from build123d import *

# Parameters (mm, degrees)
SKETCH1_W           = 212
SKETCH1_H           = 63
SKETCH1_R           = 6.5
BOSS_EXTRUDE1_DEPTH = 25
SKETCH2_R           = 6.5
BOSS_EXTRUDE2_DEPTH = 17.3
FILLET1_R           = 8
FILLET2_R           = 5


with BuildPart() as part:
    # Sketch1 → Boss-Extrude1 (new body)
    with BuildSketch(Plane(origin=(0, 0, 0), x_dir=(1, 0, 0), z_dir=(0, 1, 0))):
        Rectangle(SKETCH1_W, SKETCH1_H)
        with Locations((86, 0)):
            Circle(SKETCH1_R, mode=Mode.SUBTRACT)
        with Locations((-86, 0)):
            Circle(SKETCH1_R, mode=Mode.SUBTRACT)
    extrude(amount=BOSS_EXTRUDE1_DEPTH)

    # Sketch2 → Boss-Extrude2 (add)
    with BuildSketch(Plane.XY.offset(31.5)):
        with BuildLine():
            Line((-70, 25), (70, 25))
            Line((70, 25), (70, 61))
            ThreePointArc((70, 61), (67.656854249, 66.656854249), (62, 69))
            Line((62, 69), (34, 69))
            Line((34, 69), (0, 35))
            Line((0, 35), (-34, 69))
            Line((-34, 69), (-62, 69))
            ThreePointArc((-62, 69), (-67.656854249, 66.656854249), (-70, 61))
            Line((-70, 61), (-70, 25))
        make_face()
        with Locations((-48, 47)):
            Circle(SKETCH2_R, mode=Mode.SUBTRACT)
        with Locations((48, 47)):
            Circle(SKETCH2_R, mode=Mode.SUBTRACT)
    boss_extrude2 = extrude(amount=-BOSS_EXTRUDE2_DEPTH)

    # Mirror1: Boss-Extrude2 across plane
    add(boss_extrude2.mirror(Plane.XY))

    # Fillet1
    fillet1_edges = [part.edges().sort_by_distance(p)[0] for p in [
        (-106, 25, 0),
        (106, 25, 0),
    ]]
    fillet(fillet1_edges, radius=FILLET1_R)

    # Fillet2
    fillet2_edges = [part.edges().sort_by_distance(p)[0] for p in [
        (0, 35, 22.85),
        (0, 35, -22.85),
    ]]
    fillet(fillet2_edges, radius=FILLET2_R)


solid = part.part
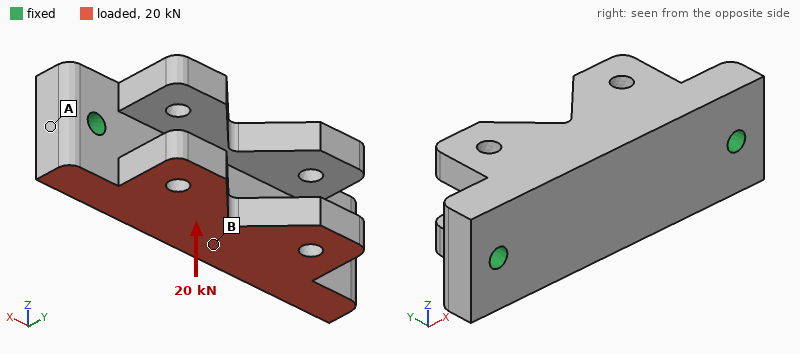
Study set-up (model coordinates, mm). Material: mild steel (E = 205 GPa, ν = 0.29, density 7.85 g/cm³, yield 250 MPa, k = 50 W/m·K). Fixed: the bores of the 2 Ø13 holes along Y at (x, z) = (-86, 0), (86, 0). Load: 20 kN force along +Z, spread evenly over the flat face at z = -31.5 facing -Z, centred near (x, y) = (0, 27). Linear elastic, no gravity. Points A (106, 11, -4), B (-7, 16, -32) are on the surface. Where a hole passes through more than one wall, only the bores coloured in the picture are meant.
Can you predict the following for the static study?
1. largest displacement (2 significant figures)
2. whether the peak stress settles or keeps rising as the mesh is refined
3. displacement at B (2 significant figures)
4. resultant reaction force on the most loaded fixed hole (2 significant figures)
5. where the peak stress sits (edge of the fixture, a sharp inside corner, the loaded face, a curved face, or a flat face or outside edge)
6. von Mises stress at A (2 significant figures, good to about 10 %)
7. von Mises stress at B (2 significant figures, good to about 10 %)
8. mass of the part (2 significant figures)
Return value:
45 µm
keeps rising
16 µm
10 kN
edge of the fixture
8.3 MPa
19 MPa
3.8 kg
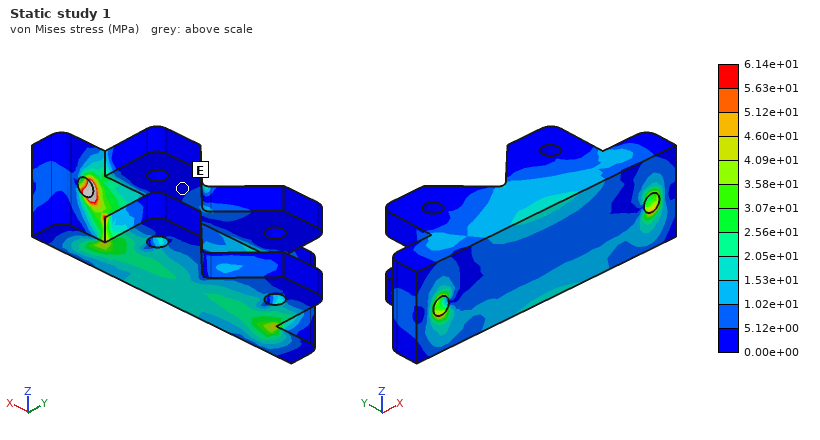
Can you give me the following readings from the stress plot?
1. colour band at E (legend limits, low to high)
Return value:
0.00e+00 to 5.12e+00 MPa
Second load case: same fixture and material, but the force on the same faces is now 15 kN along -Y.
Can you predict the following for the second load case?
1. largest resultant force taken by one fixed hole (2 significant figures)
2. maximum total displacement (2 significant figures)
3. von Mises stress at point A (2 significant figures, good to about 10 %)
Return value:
7.9 kN
38 µm
13 MPa
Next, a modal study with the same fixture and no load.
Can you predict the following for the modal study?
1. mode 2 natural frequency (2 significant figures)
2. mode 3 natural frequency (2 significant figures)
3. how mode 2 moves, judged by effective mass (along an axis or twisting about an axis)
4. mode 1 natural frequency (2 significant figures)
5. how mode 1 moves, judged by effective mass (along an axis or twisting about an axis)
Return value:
3600 Hz
4700 Hz
along Y
2700 Hz
along Z
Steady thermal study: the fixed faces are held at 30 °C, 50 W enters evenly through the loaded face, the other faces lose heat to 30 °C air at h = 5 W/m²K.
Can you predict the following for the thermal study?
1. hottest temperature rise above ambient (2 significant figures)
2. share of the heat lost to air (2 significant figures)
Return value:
19 K
4.8 %
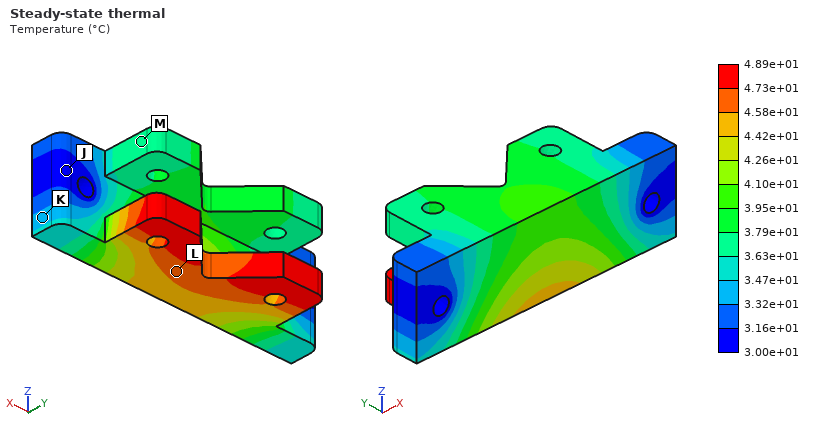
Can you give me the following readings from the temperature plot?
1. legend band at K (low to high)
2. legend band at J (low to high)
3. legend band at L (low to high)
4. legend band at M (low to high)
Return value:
3.32e+01 to 3.47e+01 °C
3.00e+01 to 3.16e+01 °C
4.58e+01 to 4.73e+01 °C
3.63e+01 to 3.79e+01 °C
